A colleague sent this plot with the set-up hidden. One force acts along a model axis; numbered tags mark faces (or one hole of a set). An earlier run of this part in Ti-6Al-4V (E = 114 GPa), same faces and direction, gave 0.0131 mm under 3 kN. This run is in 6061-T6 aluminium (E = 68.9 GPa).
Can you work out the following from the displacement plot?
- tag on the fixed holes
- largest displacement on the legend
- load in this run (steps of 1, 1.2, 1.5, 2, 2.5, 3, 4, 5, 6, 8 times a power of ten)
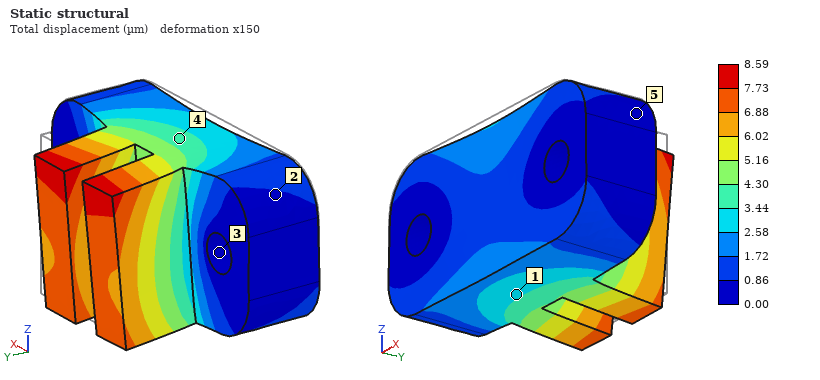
3
8.59 µm
1.2 kN
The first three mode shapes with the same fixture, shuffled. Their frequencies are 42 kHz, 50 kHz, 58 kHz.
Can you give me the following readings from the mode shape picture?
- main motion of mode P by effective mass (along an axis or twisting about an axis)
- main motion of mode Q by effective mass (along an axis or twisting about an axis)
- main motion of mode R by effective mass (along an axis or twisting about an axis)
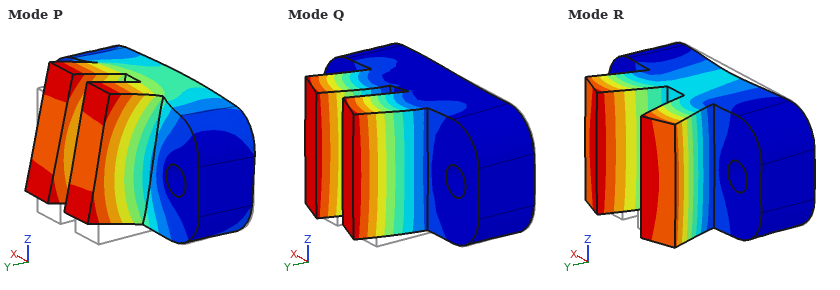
along Z
along X
along Y
